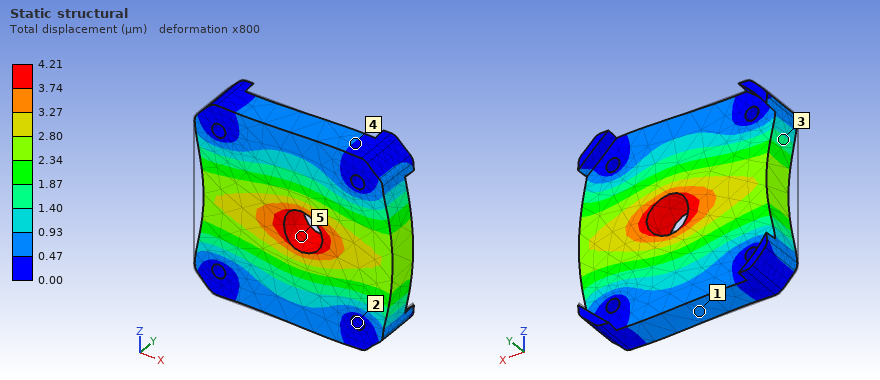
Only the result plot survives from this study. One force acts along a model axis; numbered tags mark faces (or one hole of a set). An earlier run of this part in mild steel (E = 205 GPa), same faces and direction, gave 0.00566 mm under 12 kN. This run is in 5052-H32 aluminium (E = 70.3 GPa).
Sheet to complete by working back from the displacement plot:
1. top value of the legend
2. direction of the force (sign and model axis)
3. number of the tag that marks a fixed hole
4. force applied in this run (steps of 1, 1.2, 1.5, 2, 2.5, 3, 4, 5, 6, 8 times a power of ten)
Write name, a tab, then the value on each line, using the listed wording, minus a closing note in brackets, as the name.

top value of the legend	4.21 µm
direction of the force	+X
number of the tag that marks a fixed hole	2
force applied in this run	3 kN
